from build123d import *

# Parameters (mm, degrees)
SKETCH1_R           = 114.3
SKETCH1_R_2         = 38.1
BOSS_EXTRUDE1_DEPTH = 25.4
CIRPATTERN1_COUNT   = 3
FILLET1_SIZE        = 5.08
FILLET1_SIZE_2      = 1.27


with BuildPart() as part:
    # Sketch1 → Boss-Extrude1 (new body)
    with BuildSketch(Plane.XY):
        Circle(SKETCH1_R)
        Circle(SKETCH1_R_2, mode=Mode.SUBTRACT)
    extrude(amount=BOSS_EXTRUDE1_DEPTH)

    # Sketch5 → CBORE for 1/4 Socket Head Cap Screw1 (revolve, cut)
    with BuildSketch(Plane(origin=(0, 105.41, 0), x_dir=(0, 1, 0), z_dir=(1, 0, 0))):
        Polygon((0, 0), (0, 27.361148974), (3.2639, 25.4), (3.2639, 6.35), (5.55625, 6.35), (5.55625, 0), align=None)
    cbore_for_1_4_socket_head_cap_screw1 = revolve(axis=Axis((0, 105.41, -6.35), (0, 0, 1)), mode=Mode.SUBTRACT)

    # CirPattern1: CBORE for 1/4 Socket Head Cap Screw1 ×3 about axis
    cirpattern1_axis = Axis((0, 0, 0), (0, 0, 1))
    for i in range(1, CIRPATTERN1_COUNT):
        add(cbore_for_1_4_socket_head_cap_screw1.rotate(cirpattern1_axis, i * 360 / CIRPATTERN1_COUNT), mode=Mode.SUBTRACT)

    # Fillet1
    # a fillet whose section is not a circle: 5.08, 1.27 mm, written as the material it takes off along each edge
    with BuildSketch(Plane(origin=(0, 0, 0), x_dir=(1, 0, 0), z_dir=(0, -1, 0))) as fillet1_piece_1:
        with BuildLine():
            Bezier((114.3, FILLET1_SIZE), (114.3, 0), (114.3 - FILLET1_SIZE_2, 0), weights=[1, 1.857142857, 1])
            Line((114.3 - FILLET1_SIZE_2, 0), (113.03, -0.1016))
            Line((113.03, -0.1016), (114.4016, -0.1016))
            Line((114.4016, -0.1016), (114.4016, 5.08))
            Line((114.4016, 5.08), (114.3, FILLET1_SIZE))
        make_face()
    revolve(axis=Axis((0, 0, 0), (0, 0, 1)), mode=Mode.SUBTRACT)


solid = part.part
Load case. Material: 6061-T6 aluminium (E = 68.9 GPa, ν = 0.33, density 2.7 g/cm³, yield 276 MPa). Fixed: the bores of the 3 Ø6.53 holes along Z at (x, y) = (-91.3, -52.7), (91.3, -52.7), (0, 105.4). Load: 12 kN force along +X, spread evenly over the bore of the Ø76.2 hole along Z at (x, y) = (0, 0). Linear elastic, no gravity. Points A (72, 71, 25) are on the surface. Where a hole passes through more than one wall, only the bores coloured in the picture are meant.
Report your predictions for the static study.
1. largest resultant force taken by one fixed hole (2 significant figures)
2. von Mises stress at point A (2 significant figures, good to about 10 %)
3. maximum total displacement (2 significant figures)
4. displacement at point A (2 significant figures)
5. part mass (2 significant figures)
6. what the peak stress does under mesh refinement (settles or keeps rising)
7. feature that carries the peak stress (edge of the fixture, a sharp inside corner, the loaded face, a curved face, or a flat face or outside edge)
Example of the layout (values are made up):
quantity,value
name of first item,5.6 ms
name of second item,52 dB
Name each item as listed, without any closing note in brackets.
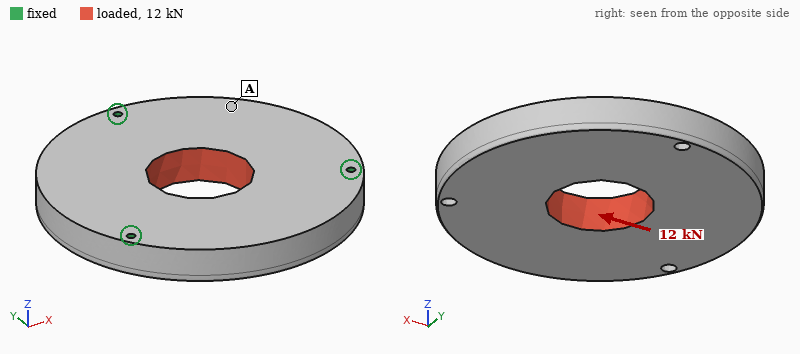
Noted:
quantity,value
largest resultant force taken by one fixed hole,4.2 kN
von Mises stress at point A,2.3 MPa
maximum total displacement,7.3 µm
displacement at point A,5.1 µm
part mass,2.5 kg
what the peak stress does under mesh refinement,keeps rising
feature that carries the peak stress,edge of the fixture
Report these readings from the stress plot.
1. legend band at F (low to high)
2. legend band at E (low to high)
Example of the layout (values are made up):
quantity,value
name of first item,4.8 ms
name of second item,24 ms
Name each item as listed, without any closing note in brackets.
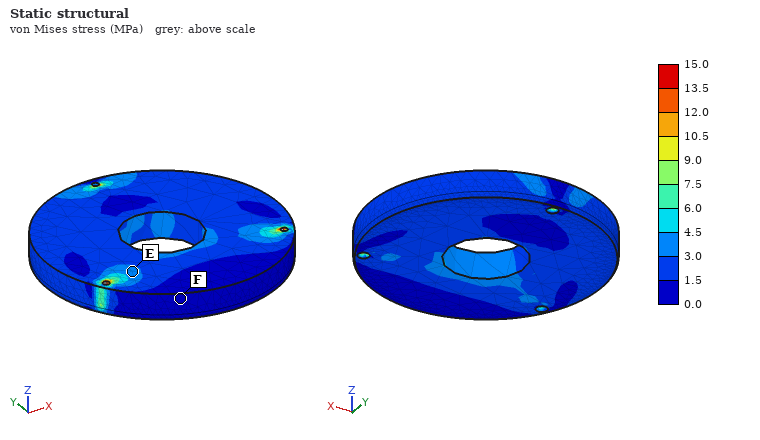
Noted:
quantity,value
legend band at F,0.0 to 1.5 MPa
legend band at E,3.0 to 4.5 MPa
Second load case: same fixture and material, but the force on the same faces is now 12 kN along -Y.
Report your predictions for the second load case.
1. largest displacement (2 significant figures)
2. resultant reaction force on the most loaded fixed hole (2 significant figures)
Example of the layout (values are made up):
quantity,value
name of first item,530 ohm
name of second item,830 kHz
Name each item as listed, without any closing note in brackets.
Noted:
quantity,value
largest displacement,7.9 µm
resultant reaction force on the most loaded fixed hole,4.1 kN
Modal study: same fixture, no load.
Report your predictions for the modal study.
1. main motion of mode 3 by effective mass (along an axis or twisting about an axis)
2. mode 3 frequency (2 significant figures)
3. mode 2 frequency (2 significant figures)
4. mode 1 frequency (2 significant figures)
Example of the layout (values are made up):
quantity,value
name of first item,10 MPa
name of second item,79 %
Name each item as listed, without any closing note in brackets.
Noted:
quantity,value
main motion of mode 3 by effective mass,along Z
mode 3 frequency,2300 Hz
mode 2 frequency,2000 Hz
mode 1 frequency,2000 Hz
